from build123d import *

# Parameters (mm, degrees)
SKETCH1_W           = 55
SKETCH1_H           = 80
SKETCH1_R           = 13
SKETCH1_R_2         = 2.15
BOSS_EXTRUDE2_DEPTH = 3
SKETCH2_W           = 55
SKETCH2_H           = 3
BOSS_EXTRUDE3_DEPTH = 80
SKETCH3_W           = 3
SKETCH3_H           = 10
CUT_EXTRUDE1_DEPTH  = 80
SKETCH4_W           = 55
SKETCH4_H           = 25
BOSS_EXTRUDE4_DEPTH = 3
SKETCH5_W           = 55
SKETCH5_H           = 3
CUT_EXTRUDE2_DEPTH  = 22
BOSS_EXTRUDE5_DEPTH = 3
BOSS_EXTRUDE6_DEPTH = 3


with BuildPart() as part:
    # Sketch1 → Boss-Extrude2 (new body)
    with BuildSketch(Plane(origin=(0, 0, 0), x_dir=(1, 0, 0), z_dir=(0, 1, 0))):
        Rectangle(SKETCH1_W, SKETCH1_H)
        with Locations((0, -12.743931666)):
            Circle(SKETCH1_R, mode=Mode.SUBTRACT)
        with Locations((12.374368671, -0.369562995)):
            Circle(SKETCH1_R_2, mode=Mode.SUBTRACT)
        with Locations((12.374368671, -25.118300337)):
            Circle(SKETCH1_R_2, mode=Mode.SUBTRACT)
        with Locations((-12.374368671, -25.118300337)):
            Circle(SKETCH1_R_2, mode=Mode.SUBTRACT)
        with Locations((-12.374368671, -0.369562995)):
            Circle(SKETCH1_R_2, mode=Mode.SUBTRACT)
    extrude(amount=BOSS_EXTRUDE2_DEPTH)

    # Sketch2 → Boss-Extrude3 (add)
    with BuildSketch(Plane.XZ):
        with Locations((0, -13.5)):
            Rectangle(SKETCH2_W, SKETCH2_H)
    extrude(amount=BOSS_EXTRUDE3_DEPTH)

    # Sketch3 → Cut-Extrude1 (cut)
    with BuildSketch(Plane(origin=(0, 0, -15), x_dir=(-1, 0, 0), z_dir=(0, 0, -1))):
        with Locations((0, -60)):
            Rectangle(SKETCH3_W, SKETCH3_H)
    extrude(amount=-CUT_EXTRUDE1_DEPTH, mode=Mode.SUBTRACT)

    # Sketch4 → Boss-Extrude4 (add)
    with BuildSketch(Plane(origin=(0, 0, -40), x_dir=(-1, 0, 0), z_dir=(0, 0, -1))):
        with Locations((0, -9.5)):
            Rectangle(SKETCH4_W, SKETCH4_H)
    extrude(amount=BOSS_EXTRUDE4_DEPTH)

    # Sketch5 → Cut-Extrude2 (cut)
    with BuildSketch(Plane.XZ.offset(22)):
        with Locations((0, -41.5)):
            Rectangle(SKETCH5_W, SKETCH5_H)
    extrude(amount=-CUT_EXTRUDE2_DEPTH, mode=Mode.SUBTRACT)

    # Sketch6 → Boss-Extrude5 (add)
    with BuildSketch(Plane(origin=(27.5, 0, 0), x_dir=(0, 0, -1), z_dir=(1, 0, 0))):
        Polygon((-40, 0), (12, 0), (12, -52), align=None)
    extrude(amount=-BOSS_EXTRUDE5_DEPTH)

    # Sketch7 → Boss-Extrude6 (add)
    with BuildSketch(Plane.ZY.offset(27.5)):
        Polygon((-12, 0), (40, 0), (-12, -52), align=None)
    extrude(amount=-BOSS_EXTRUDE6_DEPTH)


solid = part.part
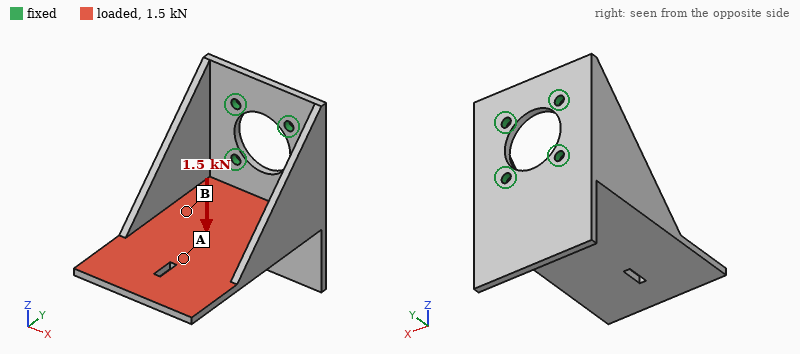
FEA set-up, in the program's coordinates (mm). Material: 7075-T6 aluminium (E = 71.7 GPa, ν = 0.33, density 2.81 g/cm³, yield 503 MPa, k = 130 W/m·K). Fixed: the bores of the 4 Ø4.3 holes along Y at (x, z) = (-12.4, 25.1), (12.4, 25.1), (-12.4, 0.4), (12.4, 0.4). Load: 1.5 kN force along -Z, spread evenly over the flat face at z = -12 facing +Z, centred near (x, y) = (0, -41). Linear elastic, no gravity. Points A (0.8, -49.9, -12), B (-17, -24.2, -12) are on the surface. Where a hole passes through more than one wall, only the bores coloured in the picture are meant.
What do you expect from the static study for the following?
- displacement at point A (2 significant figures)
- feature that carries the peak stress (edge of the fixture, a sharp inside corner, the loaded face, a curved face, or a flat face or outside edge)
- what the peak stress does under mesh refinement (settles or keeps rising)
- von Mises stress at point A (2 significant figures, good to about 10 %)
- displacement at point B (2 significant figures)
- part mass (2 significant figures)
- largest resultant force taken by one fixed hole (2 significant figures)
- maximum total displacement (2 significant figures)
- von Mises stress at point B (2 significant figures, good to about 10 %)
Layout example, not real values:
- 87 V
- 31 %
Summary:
- 0.63 mm
- edge of the fixture
- keeps rising
- 110 MPa
- 0.25 mm
- 93 g
- 1.1 kN
- 1.4 mm
- 37 MPa
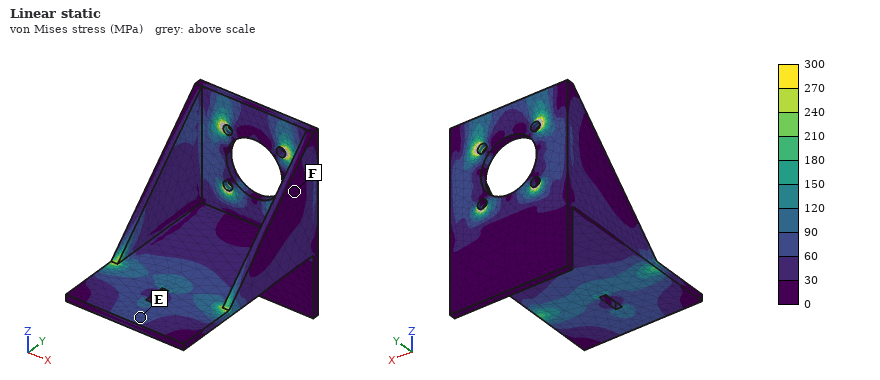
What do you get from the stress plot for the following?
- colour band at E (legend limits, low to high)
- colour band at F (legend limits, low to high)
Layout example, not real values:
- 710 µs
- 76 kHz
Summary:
- 60 to 90 MPa
- 0 to 30 MPa
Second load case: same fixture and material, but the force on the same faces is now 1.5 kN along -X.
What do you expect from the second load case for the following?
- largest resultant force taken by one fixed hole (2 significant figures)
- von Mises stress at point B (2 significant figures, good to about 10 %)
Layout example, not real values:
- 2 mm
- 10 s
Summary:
- 2.2 kN
- 43 MPa
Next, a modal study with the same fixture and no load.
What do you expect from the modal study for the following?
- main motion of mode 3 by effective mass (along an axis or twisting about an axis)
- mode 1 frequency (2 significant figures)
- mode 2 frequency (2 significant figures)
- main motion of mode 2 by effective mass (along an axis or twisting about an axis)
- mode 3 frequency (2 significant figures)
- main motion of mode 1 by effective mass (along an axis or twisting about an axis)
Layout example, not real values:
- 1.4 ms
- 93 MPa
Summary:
- along Y
- 1100 Hz
- 1200 Hz
- along X
- 2000 Hz
- along Z
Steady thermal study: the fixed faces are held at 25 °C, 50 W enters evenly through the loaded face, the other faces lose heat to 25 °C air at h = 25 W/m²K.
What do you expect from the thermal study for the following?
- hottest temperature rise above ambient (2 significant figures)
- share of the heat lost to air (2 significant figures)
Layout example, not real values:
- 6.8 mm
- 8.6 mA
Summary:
- 70 K
- 24 %
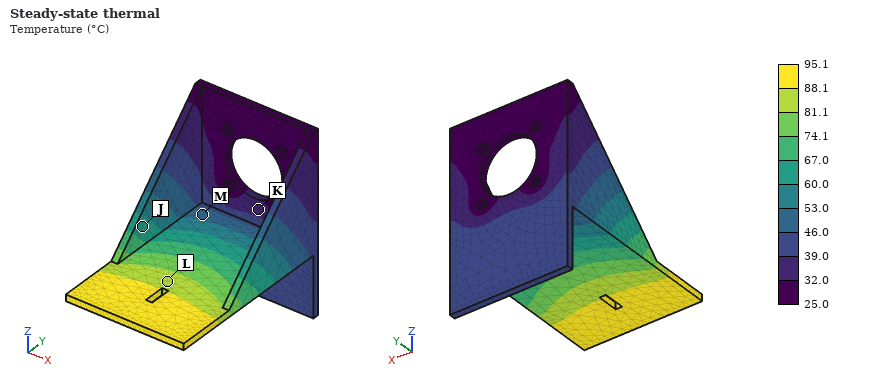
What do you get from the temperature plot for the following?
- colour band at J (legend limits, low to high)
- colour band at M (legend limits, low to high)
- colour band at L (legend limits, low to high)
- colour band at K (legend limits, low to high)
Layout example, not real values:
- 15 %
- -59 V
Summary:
- 60.0 to 67.0 °C
- 46.0 to 53.0 °C
- 81.1 to 88.1 °C
- 32.0 to 39.0 °C
